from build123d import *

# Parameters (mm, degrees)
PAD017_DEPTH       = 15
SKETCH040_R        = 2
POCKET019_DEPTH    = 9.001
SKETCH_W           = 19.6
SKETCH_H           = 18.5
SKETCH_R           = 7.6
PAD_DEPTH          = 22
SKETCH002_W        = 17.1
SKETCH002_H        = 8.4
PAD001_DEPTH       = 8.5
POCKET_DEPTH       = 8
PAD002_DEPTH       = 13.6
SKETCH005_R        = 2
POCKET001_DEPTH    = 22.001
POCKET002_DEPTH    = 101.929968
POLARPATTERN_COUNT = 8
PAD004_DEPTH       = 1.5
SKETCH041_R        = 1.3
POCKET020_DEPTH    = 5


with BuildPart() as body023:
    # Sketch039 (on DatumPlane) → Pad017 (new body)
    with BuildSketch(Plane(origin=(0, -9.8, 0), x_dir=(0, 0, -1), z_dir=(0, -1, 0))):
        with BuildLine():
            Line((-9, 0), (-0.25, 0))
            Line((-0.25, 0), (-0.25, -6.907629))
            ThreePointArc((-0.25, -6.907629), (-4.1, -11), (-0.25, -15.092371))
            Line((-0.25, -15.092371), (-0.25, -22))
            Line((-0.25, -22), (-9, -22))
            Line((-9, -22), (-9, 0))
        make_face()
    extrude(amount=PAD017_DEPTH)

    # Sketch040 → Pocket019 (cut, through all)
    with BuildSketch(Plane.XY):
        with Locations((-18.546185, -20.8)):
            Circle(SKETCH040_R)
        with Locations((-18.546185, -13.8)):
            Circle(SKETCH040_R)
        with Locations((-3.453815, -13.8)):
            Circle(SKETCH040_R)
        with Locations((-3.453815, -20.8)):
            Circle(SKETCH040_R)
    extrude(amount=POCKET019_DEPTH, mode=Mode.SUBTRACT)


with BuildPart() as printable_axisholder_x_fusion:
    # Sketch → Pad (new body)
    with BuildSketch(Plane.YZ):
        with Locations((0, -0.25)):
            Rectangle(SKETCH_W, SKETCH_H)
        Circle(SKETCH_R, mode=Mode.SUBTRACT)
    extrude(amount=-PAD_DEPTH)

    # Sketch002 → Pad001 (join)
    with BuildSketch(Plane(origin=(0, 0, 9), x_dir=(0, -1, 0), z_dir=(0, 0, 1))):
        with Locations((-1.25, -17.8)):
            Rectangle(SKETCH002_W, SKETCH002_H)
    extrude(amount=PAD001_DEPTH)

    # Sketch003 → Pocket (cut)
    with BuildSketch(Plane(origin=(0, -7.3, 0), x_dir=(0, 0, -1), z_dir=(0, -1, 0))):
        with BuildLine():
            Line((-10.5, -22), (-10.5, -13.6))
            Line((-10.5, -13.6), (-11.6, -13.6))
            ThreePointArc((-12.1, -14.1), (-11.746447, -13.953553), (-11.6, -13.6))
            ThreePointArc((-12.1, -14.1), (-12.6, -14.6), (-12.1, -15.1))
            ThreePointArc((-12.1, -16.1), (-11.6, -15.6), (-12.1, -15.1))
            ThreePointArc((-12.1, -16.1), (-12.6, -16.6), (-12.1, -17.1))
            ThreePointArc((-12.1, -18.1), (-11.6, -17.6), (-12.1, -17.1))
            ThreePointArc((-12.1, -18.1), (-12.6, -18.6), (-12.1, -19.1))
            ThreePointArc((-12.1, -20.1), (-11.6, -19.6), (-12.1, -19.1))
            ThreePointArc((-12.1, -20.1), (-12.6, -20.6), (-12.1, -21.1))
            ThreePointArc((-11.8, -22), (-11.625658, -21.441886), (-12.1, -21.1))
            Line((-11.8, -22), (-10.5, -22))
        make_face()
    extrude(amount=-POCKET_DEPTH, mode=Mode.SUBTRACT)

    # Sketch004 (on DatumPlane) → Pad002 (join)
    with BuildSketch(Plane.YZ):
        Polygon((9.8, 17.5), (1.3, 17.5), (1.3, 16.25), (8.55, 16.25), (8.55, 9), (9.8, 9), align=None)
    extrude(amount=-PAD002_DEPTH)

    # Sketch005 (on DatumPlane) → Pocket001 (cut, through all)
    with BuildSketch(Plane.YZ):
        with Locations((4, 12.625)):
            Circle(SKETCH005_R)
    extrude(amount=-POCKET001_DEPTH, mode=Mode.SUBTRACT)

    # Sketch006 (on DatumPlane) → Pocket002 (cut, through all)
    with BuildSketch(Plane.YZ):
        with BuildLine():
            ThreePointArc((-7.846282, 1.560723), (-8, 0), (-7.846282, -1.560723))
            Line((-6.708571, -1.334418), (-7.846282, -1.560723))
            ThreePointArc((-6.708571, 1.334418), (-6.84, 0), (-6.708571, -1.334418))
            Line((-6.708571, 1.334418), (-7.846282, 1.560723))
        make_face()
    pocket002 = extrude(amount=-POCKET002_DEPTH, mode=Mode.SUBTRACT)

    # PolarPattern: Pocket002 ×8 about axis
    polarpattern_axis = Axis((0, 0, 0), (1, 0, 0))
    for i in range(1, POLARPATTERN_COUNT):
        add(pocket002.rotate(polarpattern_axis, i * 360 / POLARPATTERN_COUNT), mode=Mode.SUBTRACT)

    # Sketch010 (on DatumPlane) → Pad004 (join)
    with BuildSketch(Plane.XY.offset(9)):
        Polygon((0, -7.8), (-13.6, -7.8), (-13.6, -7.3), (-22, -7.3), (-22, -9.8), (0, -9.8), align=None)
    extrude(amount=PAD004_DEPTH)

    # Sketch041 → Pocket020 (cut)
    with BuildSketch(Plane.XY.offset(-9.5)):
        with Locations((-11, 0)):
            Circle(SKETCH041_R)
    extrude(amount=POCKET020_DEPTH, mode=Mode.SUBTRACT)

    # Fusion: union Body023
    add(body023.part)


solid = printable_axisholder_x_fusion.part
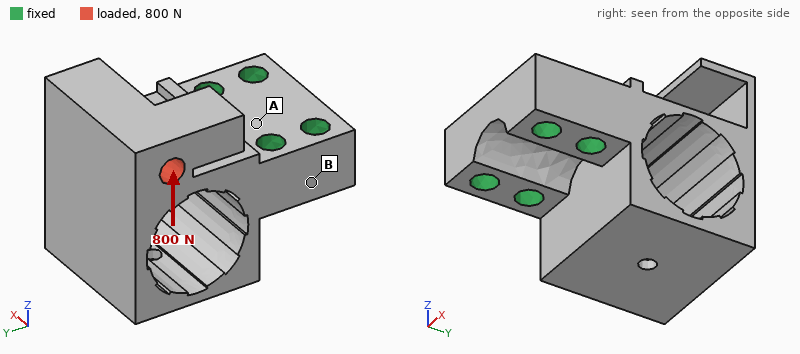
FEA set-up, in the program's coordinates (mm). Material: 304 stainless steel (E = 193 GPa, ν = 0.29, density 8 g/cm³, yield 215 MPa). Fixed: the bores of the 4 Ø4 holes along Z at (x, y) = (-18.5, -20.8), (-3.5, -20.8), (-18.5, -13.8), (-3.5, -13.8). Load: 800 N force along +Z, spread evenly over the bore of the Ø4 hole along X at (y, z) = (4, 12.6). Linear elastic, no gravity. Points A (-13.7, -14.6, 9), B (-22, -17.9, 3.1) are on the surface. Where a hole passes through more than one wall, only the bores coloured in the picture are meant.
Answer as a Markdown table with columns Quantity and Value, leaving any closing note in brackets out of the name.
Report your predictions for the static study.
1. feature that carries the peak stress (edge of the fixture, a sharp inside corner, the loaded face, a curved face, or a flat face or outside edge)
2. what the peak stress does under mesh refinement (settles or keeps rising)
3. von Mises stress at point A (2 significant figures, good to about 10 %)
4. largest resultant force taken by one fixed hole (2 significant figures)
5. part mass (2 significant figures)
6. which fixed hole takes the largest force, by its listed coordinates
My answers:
| Quantity | Value |
|---|---|
| feature that carries the peak stress | a sharp inside corner |
| what the peak stress does under mesh refinement | keeps rising |
| von Mises stress at point A | 24 MPa |
| largest resultant force taken by one fixed hole | 770 N |
| part mass | 58 g |
| which fixed hole takes the largest force, by its listed coordinates | (-18.5, -13.8) |
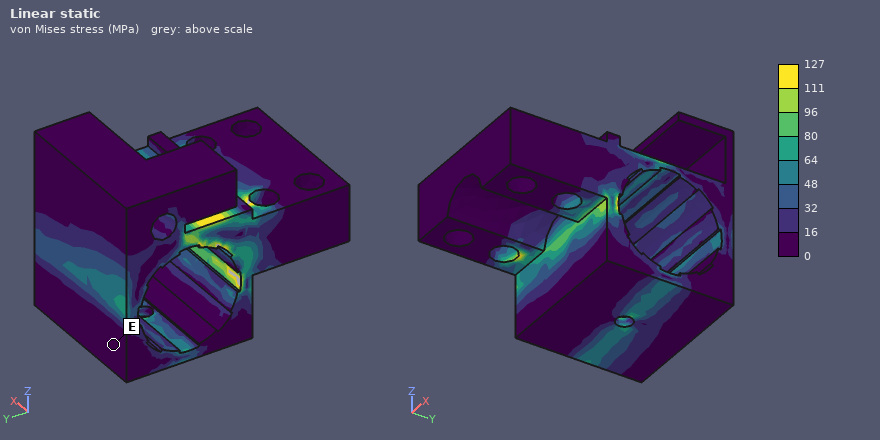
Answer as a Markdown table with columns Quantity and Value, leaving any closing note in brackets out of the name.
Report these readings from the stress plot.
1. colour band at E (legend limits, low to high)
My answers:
| Quantity | Value |
|---|---|
| colour band at E | 0 to 16 MPa |
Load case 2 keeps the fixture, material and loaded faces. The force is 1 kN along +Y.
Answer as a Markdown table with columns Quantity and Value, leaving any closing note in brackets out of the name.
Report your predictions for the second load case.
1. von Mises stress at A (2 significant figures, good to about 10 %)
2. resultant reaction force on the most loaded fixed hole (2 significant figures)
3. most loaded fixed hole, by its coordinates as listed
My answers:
| Quantity | Value |
|---|---|
| von Mises stress at A | 16 MPa |
| resultant reaction force on the most loaded fixed hole | 820 N |
| most loaded fixed hole, by its coordinates as listed | (-18.5, -13.8) |
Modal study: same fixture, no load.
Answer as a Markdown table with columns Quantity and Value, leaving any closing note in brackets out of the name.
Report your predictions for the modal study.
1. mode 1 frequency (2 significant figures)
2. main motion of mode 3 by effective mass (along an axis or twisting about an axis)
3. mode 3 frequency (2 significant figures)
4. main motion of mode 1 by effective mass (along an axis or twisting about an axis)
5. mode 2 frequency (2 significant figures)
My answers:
| Quantity | Value |
|---|---|
| mode 1 frequency | 3400 Hz |
| main motion of mode 3 by effective mass | along Z |
| mode 3 frequency | 11 kHz |
| main motion of mode 1 by effective mass | along Z |
| mode 2 frequency | 8800 Hz |
